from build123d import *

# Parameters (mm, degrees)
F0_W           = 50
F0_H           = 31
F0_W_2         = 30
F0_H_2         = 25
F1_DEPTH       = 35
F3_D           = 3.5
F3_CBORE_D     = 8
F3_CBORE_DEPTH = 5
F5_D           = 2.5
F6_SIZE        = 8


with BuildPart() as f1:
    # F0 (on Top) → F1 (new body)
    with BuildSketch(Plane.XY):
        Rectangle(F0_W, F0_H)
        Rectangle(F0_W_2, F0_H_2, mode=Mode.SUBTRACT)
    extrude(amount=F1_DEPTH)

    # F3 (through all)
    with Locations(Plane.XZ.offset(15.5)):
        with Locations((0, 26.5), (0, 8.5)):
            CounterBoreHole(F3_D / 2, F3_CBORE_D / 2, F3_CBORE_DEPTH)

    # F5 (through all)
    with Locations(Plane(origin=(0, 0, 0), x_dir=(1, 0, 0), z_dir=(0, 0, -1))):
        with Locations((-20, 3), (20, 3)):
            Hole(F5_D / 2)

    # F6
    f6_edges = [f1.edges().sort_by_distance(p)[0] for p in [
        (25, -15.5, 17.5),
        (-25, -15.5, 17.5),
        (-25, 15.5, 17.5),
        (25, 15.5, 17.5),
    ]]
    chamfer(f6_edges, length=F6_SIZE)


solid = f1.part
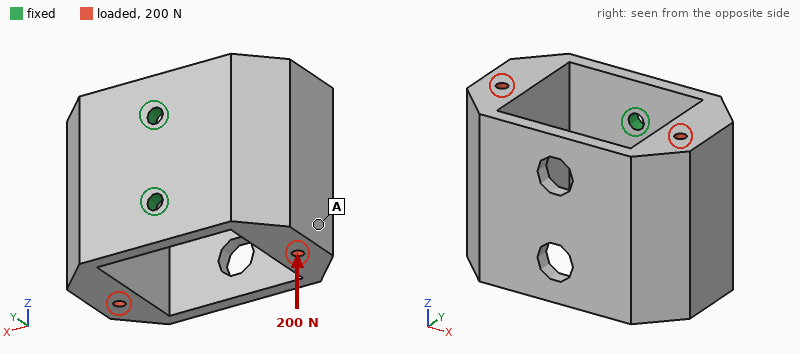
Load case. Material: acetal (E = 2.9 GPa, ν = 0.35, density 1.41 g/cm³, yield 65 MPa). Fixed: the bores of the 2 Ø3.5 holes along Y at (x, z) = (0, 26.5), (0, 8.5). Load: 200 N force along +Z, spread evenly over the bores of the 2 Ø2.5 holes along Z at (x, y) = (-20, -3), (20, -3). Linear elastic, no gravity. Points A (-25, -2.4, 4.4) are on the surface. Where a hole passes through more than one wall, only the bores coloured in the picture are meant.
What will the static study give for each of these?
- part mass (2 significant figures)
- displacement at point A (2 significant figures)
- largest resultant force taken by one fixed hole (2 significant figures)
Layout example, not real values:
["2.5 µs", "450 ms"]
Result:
["32 g", "0.49 mm", "180 N"]
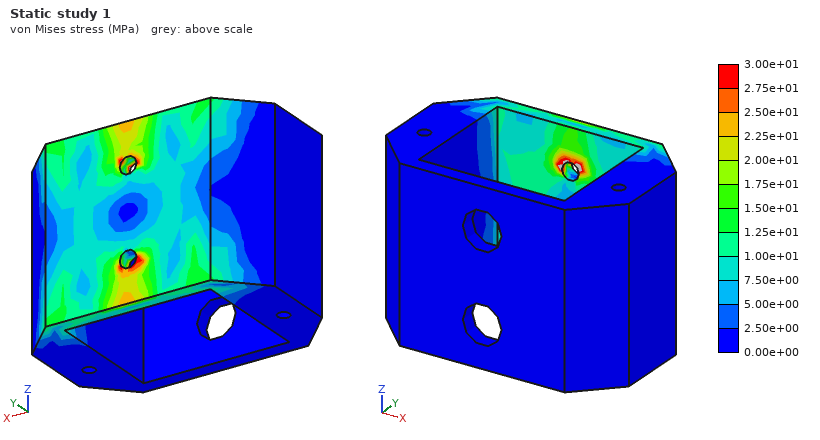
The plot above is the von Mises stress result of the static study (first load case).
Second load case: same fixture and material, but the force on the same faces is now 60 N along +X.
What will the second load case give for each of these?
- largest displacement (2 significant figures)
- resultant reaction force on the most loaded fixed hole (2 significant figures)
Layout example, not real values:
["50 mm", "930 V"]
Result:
["0.75 mm", "30 N"]
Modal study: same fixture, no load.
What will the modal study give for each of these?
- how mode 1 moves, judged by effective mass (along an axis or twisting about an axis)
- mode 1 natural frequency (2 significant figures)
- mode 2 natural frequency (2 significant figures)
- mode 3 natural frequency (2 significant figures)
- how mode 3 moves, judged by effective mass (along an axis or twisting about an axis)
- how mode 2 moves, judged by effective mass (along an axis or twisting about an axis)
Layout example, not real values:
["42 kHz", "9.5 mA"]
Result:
["along X", "280 Hz", "550 Hz", "1000 Hz", "along Y", "along Z"]
